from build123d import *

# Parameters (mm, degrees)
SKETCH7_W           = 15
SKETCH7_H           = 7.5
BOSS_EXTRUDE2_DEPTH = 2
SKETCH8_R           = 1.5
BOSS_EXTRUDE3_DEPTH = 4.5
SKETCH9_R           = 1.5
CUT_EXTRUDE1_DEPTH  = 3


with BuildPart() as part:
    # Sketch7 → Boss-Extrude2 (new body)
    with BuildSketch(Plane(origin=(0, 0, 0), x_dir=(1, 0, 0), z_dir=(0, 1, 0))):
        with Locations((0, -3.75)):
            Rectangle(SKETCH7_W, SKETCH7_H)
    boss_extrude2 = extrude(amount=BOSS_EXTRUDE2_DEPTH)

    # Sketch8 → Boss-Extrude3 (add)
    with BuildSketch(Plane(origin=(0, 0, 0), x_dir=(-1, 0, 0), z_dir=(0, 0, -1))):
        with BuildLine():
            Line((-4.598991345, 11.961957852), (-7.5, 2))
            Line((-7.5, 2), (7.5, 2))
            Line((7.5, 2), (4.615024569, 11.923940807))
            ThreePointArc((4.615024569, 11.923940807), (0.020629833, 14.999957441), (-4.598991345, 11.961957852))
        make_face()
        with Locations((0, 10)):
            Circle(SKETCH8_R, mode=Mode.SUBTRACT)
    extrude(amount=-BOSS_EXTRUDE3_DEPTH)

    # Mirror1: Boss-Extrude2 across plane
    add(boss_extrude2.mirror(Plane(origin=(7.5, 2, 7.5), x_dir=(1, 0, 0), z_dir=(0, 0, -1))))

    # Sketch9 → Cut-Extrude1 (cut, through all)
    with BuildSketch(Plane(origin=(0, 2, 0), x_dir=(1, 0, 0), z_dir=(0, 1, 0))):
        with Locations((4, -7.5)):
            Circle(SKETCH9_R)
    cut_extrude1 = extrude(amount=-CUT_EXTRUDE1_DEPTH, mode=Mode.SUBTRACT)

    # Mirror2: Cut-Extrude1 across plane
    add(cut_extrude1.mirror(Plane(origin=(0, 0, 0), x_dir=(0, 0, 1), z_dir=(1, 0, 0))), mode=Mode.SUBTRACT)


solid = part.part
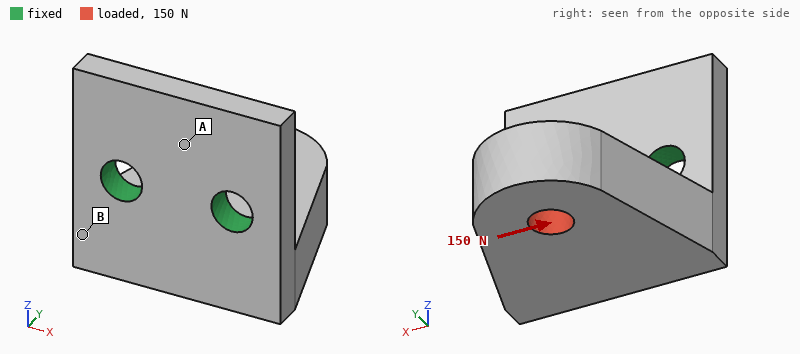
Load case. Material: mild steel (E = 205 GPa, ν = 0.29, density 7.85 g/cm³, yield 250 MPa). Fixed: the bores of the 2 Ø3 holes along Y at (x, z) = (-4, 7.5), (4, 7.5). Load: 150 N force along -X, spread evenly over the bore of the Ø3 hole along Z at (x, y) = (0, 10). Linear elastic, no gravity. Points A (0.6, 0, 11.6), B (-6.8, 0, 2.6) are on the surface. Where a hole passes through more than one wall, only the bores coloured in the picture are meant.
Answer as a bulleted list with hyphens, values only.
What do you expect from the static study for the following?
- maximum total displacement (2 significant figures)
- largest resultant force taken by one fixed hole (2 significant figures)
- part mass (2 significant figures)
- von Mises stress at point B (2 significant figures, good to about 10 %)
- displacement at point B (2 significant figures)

- 4.3 µm
- 170 N
- 8.0 g
- 14 MPa
- 1.6 µm
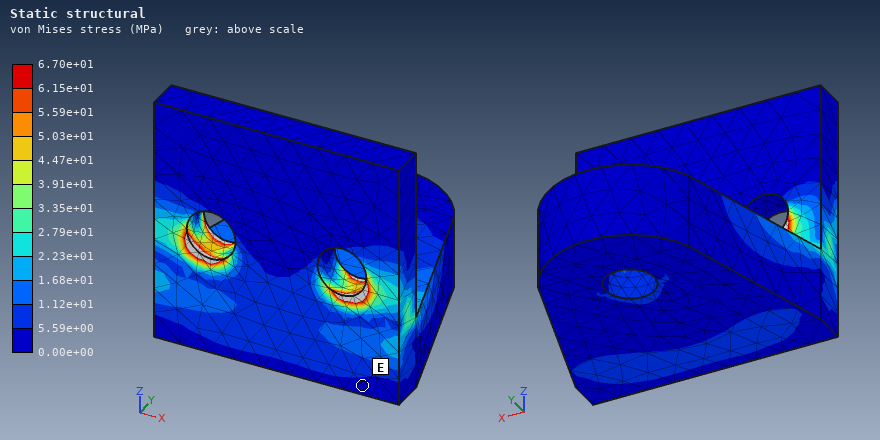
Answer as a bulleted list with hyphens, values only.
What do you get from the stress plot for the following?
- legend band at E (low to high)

- 0.00e+00 to 5.59e+00 MPa
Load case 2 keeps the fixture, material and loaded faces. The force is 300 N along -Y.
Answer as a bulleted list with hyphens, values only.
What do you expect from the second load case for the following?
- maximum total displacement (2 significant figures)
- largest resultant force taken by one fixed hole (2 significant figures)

- 20 µm
- 150 N
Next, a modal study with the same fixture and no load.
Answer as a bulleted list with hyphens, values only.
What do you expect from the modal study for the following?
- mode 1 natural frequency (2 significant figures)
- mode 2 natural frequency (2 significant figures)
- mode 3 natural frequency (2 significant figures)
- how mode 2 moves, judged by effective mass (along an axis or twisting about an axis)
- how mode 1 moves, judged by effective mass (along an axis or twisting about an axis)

- 7200 Hz
- 19 kHz
- 35 kHz
- along X
- along Z
